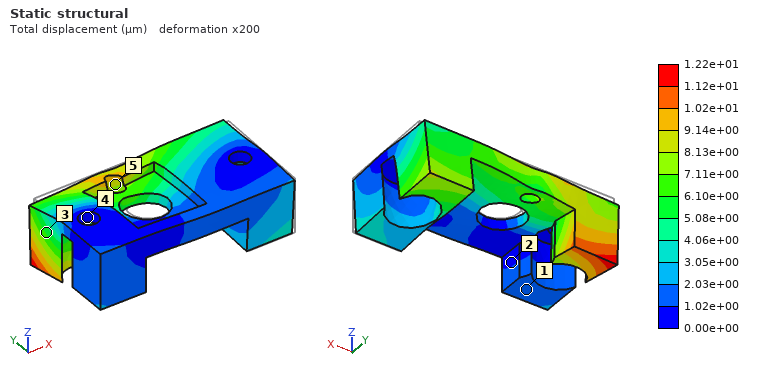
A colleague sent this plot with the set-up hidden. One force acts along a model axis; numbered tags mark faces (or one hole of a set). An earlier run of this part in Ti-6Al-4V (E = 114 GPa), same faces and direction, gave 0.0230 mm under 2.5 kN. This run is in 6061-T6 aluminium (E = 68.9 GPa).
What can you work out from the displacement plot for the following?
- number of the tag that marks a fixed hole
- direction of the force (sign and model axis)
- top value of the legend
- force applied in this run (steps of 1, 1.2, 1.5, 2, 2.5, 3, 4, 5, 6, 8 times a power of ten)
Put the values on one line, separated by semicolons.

4; -X; 1.22e+01 µm; 800 N
